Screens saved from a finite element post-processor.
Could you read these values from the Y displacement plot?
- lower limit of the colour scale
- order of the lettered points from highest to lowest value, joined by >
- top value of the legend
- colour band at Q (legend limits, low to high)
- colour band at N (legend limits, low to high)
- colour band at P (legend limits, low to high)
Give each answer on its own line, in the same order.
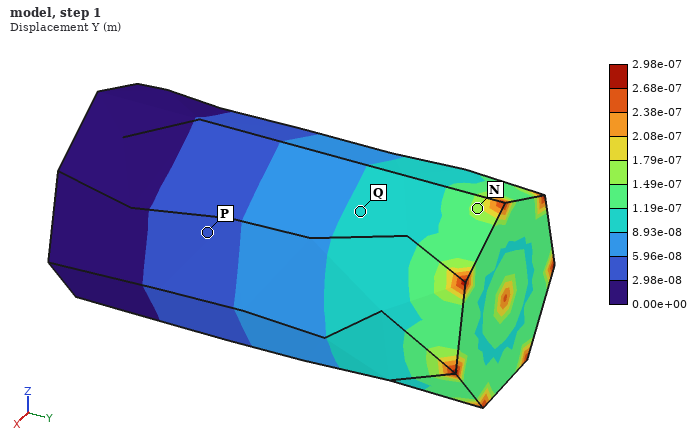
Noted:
0.00e+00 m
N > Q > P
2.98e-07 m
8.93e-08 to 1.19e-07 m
1.49e-07 to 1.79e-07 m
2.98e-08 to 5.96e-08 m
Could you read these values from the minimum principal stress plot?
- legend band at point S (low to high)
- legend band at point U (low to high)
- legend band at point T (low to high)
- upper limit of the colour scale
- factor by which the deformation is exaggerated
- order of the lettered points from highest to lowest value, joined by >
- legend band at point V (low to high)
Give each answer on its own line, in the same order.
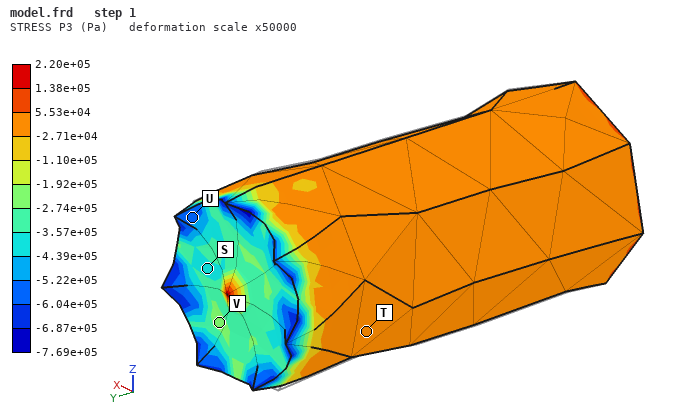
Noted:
-4.39e+05 to -3.57e+05 Pa
-6.04e+05 to -5.22e+05 Pa
-2.71e+04 to 5.53e+04 Pa
2.20e+05 Pa
50000
T > V > S > U
-2.74e+05 to -1.92e+05 Pa
